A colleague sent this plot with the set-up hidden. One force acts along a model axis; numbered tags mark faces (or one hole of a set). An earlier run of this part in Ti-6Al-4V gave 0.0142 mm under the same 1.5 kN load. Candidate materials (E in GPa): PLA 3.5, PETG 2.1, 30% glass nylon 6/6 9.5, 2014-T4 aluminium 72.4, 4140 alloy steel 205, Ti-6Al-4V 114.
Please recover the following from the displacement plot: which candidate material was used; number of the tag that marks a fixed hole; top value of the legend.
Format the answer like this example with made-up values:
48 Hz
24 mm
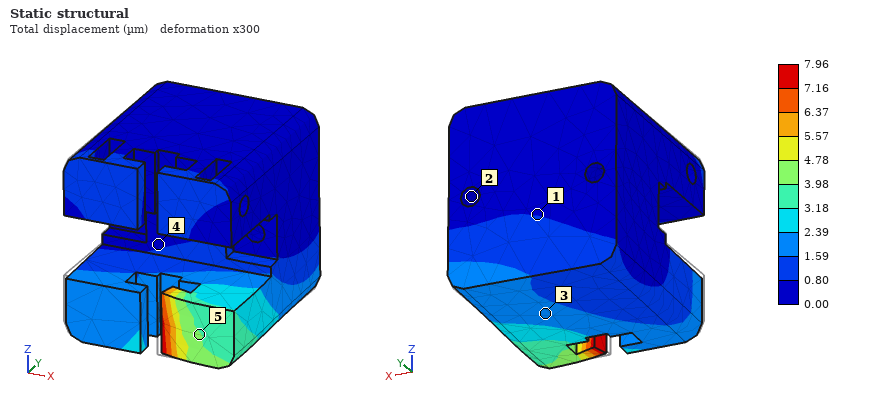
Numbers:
4140 alloy steel
2
7.96 µm
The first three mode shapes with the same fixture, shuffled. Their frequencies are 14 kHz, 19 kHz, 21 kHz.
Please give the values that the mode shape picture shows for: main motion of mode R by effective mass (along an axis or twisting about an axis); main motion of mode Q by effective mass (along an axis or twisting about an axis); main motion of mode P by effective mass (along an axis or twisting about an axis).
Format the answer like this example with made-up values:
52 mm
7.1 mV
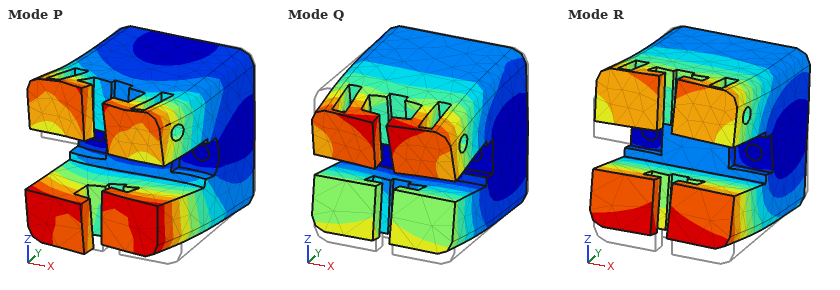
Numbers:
along Z
along Y
along X
